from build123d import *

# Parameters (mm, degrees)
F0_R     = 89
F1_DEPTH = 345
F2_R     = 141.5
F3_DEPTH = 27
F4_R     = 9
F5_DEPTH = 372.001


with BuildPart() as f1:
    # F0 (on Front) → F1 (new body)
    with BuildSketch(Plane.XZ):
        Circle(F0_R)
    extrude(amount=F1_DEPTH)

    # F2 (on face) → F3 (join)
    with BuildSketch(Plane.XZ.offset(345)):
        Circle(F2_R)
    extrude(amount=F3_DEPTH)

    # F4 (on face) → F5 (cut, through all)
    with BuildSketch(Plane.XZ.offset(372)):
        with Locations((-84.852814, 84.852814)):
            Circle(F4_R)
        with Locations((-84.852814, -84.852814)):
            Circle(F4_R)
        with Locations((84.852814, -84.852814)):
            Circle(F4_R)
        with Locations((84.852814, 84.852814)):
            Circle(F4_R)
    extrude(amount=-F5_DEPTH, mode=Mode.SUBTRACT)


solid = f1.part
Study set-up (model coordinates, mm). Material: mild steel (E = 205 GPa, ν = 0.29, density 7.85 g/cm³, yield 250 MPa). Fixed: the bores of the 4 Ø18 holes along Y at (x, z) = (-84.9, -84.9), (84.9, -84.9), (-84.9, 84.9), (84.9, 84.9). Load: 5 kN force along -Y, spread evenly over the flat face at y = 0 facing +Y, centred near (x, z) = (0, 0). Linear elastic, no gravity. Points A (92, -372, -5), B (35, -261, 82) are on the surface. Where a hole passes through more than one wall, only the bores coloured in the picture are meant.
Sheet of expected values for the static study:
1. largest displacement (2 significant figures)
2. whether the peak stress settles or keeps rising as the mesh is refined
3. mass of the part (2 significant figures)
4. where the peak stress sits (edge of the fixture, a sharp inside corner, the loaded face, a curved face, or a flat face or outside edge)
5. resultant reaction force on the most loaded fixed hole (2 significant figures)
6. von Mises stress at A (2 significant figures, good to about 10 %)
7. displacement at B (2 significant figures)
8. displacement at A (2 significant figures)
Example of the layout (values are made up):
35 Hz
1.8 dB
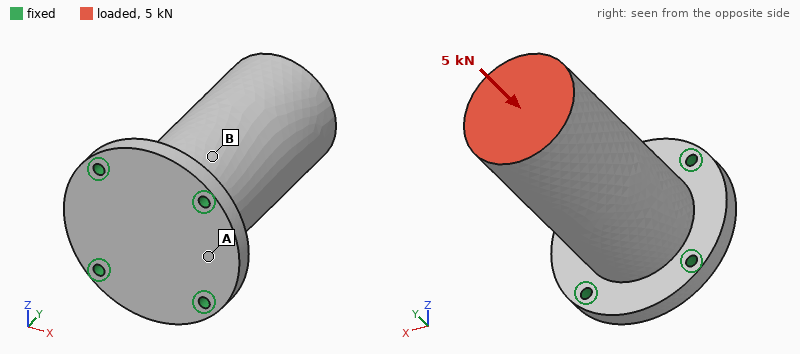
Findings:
1.1 µm
keeps rising
81 kg
edge of the fixture
1.3 kN
0.61 MPa
0.82 µm
0.69 µm
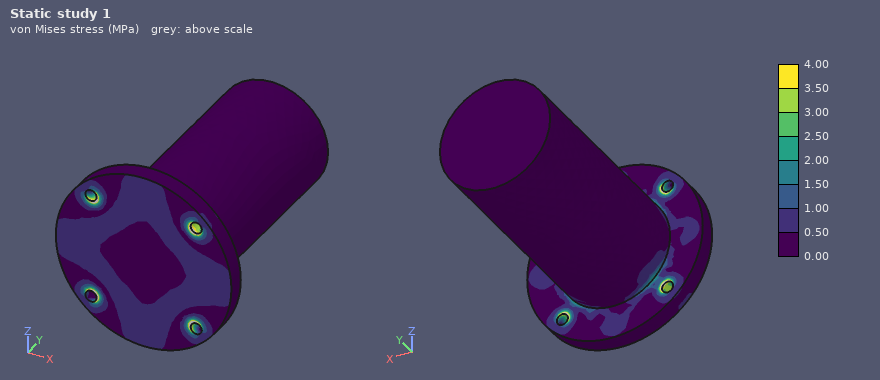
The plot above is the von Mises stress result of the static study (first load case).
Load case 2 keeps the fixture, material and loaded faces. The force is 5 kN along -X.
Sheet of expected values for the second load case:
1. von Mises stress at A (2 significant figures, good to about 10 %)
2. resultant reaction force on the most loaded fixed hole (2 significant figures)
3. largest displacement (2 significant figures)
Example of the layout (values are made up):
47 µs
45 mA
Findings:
4.1 MPa
5.9 kN
25 µm
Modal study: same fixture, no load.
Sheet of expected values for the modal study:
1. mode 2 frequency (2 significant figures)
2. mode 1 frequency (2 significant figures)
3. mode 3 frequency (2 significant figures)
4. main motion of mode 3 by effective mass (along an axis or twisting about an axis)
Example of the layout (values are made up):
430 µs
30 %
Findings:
490 Hz
490 Hz
1400 Hz
along Y
